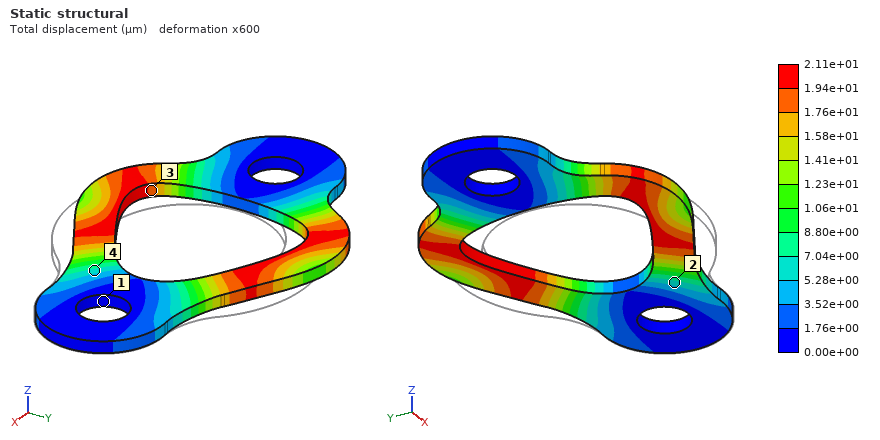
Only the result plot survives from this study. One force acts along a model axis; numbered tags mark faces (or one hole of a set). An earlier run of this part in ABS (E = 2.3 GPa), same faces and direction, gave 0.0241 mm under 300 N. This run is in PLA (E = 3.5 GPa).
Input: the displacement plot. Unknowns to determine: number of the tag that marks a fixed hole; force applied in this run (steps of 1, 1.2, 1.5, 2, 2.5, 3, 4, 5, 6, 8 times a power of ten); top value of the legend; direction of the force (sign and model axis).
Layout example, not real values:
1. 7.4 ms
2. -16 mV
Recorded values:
1. 1
2. 400 N
3. 2.11e+01 µm
4. -X
